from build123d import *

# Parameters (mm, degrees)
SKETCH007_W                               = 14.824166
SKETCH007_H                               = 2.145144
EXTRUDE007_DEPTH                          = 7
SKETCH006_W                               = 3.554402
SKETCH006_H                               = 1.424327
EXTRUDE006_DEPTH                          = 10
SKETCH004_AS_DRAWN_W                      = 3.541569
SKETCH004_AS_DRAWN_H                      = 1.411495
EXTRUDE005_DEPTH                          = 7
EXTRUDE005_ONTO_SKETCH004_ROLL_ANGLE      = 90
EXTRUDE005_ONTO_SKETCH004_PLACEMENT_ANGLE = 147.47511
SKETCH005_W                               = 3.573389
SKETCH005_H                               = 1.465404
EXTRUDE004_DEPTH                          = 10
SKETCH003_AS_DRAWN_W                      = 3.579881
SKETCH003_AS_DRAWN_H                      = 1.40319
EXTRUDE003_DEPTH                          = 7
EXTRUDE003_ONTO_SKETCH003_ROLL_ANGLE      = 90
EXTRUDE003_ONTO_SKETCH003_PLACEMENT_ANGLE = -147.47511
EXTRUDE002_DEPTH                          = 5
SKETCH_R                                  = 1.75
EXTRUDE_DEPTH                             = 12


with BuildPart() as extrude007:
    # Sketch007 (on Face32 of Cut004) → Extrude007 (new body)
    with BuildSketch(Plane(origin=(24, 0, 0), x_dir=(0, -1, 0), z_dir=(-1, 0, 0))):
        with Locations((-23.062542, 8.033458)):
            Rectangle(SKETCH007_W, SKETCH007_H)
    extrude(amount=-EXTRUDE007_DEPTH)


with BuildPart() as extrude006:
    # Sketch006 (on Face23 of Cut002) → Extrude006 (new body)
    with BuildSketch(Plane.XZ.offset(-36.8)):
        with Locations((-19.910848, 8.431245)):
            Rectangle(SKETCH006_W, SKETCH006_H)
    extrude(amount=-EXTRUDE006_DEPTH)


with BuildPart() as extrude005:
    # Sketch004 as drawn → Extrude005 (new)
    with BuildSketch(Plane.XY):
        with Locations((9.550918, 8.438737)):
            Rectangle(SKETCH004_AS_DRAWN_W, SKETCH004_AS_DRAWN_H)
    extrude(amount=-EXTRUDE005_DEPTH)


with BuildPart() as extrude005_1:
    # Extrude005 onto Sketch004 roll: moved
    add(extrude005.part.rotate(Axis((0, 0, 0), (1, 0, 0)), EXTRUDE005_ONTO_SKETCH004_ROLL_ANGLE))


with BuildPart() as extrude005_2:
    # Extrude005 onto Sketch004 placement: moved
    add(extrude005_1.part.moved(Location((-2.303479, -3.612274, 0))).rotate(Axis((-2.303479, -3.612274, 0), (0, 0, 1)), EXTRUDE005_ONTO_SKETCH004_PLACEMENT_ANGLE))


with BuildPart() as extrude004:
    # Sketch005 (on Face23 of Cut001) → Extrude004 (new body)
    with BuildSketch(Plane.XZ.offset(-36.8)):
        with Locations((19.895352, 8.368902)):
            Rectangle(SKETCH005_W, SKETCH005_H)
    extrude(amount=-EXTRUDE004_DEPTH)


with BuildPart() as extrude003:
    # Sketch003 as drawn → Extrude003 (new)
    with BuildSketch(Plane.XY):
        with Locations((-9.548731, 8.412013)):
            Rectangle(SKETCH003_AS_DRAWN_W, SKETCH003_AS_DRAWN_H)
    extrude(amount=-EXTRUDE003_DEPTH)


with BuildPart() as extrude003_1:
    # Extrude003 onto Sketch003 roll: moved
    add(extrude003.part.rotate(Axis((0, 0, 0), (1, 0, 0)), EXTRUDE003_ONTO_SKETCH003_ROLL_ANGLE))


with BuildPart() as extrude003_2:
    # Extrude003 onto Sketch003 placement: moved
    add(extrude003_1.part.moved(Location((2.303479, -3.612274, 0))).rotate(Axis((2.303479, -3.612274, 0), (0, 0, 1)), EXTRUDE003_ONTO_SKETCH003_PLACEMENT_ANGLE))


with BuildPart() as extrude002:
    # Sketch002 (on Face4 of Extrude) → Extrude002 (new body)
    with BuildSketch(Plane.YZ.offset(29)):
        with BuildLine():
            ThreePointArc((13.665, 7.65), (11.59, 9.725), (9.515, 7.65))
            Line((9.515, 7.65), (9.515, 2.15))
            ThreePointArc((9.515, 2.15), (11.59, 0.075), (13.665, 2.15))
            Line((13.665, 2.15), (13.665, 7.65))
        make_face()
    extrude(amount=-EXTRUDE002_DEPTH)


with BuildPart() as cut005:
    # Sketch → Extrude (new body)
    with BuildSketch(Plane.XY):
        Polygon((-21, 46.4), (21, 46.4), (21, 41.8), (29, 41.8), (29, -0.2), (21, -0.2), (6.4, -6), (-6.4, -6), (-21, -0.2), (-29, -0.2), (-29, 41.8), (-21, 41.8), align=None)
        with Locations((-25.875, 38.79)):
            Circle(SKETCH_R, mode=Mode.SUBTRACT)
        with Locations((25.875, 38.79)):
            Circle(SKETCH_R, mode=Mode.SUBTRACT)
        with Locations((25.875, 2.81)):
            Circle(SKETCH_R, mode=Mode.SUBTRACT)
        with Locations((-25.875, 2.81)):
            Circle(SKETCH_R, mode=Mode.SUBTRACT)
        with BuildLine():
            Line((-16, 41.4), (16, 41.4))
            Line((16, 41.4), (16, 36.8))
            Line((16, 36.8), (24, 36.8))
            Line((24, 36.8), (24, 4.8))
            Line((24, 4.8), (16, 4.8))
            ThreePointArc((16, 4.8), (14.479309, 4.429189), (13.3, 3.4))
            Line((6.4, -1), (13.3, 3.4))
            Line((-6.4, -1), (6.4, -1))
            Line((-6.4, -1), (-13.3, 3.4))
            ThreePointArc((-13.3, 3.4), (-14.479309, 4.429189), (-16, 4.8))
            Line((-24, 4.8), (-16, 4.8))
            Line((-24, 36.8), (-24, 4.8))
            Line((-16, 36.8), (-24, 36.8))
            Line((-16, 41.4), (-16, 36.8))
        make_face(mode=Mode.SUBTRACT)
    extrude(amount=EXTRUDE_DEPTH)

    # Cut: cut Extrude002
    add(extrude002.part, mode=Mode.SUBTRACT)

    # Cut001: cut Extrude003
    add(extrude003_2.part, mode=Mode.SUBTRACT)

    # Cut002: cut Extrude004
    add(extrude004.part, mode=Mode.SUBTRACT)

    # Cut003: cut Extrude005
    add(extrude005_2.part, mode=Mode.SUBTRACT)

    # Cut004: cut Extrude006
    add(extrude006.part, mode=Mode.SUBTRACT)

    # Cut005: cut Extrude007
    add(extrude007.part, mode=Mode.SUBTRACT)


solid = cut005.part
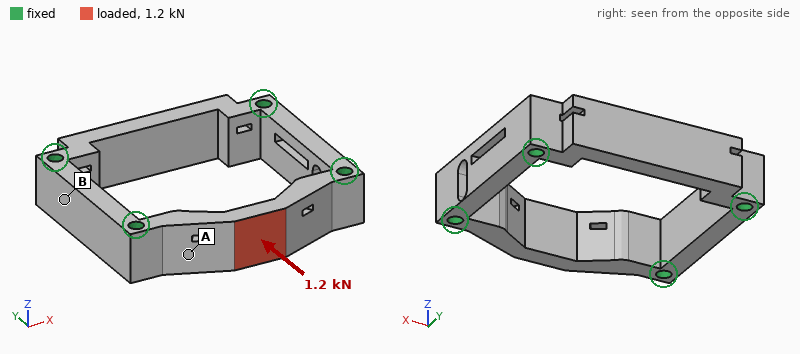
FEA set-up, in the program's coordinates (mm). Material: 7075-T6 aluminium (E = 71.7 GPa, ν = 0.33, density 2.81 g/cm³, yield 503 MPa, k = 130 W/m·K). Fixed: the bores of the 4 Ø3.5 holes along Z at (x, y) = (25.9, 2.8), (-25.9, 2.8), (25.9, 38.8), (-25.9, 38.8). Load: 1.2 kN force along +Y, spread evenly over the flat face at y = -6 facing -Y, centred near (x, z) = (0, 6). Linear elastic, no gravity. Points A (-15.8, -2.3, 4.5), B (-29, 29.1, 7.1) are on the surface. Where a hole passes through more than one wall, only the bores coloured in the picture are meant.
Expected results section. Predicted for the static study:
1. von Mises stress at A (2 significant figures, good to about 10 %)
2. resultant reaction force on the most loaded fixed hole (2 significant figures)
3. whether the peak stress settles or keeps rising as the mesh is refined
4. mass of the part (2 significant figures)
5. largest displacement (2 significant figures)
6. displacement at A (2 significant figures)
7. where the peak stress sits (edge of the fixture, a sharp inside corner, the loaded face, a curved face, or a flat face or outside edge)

24 MPa
1.4 kN
keeps rising
30 g
30 µm
12 µm
edge of the fixture
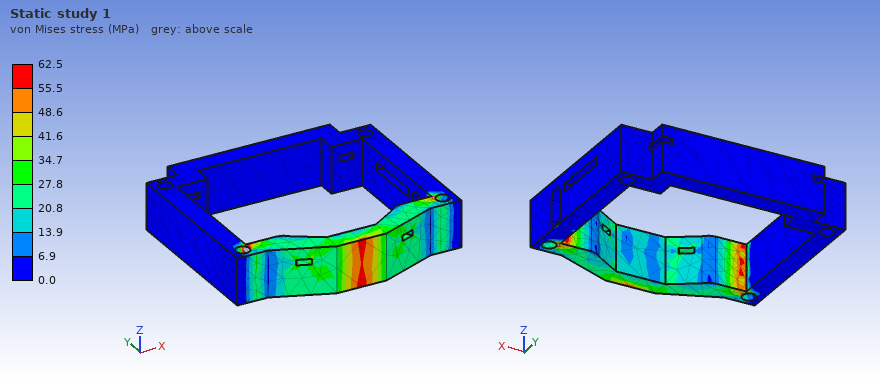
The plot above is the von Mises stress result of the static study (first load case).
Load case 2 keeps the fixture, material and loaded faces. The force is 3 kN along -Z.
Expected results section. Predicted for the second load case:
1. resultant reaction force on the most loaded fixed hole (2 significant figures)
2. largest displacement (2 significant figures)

1.5 kN
0.15 mm
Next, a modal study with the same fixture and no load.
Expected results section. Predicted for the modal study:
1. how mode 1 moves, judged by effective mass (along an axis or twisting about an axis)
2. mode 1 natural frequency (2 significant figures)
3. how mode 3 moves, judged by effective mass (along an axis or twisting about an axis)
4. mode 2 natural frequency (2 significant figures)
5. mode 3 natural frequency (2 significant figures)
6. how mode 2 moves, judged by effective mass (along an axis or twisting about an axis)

along Y
13 kHz
along Y
15 kHz
16 kHz
along Z
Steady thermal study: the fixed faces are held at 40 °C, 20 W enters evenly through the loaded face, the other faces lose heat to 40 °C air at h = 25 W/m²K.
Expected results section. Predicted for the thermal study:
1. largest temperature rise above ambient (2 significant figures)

29 K
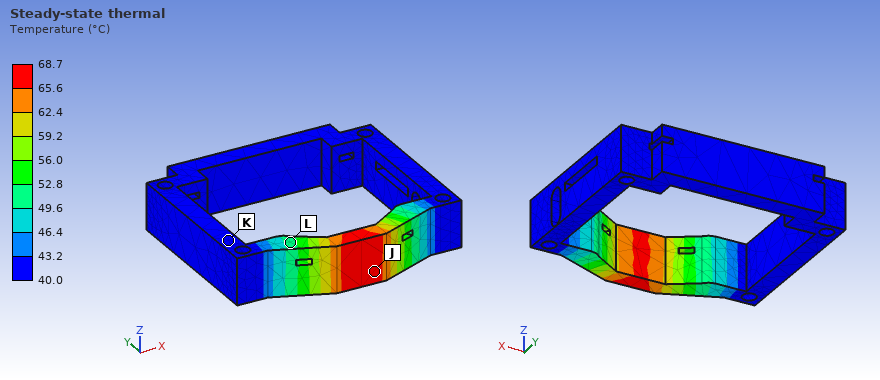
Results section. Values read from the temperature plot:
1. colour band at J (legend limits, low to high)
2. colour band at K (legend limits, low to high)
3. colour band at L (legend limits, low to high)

65.6 to 68.7 °C
40.0 to 43.2 °C
49.6 to 52.8 °C
